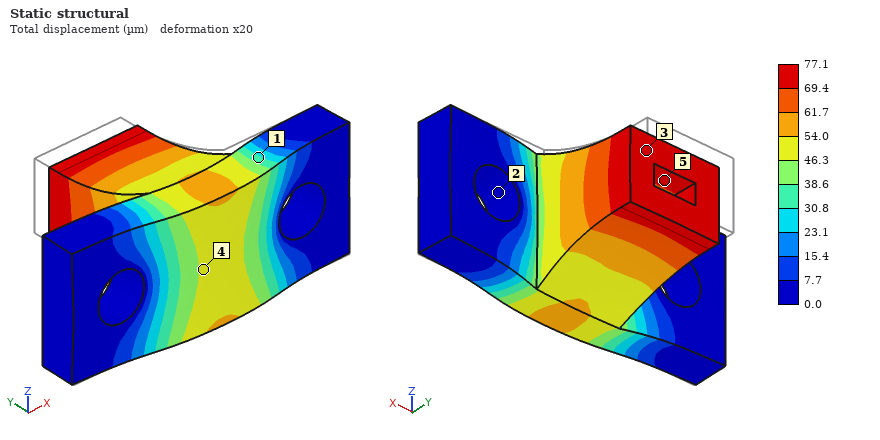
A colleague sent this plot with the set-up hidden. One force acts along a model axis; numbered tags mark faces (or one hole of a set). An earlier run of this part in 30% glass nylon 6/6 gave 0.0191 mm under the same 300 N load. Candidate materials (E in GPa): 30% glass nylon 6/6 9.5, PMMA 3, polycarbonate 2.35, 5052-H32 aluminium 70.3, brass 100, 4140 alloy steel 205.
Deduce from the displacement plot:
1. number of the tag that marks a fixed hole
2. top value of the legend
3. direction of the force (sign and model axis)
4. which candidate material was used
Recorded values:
2
77.1 µm
-Y
polycarbonate
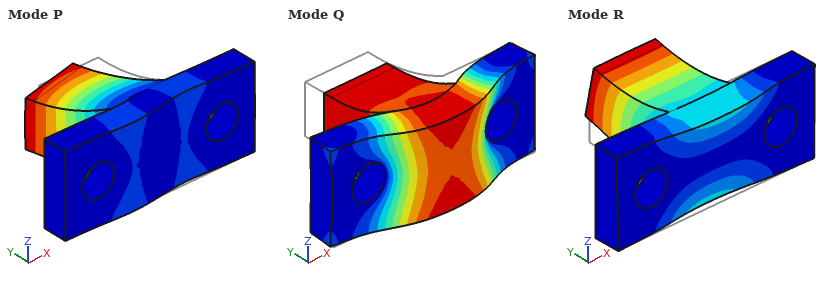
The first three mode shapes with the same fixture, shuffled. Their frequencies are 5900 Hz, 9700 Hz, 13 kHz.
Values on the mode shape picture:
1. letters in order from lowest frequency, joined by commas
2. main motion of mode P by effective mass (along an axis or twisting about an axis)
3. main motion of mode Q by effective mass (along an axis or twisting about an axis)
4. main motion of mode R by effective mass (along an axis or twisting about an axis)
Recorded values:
R, P, Q
along X
along Y
along Z
